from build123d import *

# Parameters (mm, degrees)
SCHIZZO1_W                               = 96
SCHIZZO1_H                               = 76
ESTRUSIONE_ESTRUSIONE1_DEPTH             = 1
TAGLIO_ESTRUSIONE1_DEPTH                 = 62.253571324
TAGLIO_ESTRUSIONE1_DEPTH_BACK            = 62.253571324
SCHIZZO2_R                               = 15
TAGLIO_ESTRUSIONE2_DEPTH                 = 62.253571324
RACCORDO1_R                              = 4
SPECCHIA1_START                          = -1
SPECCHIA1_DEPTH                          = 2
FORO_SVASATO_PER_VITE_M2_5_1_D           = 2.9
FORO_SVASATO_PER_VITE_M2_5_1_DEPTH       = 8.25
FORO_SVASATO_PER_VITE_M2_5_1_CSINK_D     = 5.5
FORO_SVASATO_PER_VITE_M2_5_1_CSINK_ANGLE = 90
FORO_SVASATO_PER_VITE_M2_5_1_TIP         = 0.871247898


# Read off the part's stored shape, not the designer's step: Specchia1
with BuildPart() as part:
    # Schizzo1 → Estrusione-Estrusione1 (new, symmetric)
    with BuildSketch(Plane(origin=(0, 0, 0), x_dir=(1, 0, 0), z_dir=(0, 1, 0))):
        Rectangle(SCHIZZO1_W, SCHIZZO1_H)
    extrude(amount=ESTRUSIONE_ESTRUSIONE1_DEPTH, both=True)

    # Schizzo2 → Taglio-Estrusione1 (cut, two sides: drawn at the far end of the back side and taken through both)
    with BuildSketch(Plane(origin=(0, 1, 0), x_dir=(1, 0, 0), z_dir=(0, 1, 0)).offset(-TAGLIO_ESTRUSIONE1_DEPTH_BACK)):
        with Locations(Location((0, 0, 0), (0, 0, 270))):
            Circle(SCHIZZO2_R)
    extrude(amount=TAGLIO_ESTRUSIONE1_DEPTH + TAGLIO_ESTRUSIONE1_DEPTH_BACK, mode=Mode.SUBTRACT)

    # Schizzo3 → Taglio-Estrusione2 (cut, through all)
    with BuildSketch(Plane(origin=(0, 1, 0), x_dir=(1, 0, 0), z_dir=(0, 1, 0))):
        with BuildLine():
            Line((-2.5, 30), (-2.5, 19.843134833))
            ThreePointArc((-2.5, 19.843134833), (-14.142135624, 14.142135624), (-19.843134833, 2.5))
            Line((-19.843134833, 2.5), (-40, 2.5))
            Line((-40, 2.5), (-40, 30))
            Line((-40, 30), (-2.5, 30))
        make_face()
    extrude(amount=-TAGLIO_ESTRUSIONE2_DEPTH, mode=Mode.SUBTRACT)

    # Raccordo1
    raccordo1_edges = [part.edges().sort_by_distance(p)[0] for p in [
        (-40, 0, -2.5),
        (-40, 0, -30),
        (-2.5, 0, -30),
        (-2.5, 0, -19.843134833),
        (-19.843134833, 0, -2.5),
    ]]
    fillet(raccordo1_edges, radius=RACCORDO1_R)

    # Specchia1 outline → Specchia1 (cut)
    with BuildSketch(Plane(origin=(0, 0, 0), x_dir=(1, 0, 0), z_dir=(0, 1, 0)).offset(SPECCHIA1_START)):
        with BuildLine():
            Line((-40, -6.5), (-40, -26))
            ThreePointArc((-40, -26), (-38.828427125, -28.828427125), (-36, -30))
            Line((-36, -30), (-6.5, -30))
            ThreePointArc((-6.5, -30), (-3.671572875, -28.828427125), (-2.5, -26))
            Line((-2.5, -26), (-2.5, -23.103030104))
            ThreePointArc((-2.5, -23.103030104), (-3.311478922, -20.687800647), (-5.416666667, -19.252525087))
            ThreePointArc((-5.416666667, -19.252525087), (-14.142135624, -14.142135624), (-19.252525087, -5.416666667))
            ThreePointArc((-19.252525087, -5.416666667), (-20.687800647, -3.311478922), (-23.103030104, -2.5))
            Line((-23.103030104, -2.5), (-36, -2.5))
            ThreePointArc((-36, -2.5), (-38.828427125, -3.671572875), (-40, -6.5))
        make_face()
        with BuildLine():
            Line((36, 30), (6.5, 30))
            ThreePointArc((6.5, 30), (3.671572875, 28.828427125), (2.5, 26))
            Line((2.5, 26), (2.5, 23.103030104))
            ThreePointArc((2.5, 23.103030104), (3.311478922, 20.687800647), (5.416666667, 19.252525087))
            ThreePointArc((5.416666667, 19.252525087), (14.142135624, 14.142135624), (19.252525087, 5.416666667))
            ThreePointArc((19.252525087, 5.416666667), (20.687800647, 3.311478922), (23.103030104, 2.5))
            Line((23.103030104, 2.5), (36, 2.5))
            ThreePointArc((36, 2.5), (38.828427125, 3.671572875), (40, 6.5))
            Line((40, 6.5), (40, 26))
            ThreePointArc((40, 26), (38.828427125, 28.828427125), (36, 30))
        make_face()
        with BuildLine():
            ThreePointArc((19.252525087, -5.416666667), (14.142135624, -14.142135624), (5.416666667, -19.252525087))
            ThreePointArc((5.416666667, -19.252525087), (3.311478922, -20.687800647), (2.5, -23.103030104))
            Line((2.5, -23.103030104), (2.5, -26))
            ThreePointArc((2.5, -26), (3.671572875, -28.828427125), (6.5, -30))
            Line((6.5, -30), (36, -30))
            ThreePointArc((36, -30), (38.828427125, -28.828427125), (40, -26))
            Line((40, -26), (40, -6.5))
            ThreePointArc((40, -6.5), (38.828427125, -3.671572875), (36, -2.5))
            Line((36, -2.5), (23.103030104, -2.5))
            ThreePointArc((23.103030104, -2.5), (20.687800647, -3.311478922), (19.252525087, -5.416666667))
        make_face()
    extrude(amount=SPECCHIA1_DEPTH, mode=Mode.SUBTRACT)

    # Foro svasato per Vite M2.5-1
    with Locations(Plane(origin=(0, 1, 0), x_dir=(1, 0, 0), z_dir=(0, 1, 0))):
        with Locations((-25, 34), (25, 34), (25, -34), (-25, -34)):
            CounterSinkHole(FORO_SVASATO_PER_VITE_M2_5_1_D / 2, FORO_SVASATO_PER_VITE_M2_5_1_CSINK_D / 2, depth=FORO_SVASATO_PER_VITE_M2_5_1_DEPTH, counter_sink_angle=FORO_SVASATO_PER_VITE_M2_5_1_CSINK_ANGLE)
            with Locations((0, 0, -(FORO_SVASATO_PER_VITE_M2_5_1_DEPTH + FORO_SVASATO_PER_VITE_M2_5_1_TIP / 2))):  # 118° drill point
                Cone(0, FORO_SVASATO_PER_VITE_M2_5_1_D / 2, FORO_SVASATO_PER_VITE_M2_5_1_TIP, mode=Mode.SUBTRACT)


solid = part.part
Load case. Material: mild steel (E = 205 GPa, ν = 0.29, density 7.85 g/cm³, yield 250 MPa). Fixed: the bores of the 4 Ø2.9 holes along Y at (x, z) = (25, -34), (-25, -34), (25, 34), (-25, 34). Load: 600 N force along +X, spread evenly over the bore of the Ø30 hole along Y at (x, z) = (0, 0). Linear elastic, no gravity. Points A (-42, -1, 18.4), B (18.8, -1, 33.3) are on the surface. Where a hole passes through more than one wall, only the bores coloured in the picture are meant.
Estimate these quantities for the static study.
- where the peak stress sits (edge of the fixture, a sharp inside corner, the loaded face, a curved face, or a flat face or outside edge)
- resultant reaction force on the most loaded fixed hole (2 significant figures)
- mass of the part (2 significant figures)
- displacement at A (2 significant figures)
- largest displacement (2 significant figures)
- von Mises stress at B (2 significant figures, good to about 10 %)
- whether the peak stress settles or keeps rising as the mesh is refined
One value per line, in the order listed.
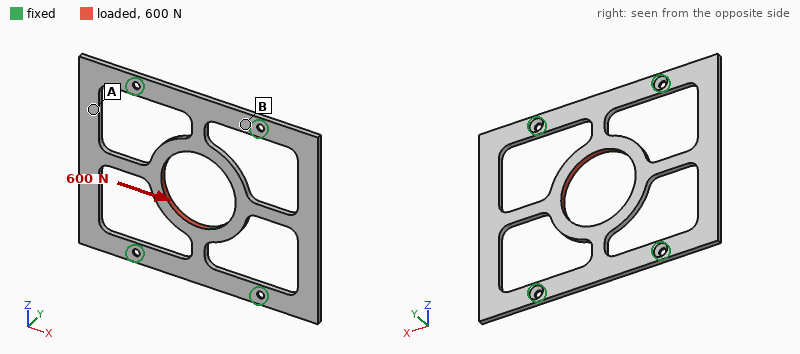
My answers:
edge of the fixture
150 N
53 g
5.8 µm
15 µm
14 MPa
keeps rising
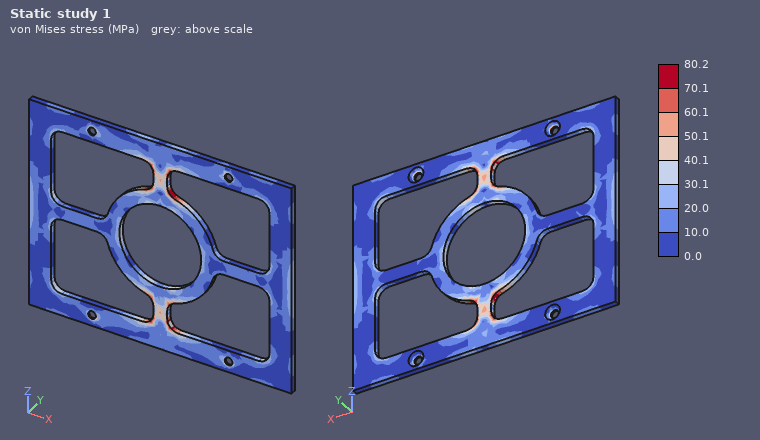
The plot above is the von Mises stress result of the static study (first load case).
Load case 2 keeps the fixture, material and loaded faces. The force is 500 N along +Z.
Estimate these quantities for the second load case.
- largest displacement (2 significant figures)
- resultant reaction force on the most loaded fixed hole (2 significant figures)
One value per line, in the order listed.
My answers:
16 µm
130 N
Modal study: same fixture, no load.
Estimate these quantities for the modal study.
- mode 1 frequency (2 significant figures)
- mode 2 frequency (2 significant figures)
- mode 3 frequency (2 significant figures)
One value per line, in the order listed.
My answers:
1100 Hz
1100 Hz
1500 Hz
